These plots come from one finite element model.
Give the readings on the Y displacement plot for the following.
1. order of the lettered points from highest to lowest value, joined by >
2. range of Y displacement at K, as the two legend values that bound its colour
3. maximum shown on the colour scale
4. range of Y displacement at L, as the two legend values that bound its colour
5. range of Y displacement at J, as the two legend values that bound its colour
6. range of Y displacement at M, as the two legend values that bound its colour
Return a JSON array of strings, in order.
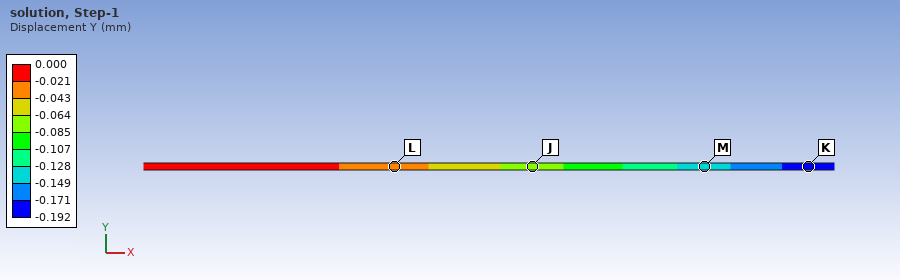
["L > J > M > K", "-0.192 to -0.171 mm", "0.000 mm", "-0.043 to -0.021 mm", "-0.085 to -0.064 mm", "-0.149 to -0.128 mm"]
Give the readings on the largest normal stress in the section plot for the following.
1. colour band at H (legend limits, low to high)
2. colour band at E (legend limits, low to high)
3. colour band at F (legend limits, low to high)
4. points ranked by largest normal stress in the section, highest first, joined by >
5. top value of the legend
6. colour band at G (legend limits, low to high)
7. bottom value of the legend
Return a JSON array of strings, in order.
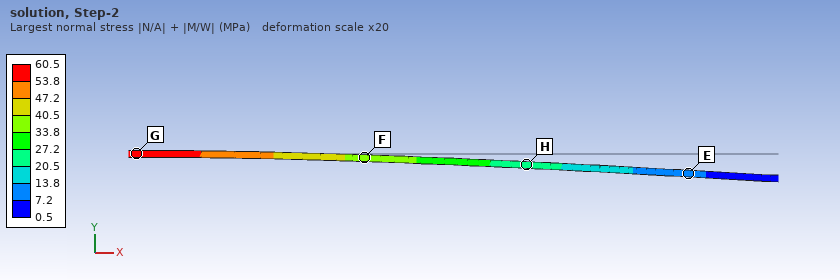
["20.5 to 27.2 MPa", "7.2 to 13.8 MPa", "33.8 to 40.5 MPa", "G > F > H > E", "60.5 MPa", "53.8 to 60.5 MPa", "0.5 MPa"]
